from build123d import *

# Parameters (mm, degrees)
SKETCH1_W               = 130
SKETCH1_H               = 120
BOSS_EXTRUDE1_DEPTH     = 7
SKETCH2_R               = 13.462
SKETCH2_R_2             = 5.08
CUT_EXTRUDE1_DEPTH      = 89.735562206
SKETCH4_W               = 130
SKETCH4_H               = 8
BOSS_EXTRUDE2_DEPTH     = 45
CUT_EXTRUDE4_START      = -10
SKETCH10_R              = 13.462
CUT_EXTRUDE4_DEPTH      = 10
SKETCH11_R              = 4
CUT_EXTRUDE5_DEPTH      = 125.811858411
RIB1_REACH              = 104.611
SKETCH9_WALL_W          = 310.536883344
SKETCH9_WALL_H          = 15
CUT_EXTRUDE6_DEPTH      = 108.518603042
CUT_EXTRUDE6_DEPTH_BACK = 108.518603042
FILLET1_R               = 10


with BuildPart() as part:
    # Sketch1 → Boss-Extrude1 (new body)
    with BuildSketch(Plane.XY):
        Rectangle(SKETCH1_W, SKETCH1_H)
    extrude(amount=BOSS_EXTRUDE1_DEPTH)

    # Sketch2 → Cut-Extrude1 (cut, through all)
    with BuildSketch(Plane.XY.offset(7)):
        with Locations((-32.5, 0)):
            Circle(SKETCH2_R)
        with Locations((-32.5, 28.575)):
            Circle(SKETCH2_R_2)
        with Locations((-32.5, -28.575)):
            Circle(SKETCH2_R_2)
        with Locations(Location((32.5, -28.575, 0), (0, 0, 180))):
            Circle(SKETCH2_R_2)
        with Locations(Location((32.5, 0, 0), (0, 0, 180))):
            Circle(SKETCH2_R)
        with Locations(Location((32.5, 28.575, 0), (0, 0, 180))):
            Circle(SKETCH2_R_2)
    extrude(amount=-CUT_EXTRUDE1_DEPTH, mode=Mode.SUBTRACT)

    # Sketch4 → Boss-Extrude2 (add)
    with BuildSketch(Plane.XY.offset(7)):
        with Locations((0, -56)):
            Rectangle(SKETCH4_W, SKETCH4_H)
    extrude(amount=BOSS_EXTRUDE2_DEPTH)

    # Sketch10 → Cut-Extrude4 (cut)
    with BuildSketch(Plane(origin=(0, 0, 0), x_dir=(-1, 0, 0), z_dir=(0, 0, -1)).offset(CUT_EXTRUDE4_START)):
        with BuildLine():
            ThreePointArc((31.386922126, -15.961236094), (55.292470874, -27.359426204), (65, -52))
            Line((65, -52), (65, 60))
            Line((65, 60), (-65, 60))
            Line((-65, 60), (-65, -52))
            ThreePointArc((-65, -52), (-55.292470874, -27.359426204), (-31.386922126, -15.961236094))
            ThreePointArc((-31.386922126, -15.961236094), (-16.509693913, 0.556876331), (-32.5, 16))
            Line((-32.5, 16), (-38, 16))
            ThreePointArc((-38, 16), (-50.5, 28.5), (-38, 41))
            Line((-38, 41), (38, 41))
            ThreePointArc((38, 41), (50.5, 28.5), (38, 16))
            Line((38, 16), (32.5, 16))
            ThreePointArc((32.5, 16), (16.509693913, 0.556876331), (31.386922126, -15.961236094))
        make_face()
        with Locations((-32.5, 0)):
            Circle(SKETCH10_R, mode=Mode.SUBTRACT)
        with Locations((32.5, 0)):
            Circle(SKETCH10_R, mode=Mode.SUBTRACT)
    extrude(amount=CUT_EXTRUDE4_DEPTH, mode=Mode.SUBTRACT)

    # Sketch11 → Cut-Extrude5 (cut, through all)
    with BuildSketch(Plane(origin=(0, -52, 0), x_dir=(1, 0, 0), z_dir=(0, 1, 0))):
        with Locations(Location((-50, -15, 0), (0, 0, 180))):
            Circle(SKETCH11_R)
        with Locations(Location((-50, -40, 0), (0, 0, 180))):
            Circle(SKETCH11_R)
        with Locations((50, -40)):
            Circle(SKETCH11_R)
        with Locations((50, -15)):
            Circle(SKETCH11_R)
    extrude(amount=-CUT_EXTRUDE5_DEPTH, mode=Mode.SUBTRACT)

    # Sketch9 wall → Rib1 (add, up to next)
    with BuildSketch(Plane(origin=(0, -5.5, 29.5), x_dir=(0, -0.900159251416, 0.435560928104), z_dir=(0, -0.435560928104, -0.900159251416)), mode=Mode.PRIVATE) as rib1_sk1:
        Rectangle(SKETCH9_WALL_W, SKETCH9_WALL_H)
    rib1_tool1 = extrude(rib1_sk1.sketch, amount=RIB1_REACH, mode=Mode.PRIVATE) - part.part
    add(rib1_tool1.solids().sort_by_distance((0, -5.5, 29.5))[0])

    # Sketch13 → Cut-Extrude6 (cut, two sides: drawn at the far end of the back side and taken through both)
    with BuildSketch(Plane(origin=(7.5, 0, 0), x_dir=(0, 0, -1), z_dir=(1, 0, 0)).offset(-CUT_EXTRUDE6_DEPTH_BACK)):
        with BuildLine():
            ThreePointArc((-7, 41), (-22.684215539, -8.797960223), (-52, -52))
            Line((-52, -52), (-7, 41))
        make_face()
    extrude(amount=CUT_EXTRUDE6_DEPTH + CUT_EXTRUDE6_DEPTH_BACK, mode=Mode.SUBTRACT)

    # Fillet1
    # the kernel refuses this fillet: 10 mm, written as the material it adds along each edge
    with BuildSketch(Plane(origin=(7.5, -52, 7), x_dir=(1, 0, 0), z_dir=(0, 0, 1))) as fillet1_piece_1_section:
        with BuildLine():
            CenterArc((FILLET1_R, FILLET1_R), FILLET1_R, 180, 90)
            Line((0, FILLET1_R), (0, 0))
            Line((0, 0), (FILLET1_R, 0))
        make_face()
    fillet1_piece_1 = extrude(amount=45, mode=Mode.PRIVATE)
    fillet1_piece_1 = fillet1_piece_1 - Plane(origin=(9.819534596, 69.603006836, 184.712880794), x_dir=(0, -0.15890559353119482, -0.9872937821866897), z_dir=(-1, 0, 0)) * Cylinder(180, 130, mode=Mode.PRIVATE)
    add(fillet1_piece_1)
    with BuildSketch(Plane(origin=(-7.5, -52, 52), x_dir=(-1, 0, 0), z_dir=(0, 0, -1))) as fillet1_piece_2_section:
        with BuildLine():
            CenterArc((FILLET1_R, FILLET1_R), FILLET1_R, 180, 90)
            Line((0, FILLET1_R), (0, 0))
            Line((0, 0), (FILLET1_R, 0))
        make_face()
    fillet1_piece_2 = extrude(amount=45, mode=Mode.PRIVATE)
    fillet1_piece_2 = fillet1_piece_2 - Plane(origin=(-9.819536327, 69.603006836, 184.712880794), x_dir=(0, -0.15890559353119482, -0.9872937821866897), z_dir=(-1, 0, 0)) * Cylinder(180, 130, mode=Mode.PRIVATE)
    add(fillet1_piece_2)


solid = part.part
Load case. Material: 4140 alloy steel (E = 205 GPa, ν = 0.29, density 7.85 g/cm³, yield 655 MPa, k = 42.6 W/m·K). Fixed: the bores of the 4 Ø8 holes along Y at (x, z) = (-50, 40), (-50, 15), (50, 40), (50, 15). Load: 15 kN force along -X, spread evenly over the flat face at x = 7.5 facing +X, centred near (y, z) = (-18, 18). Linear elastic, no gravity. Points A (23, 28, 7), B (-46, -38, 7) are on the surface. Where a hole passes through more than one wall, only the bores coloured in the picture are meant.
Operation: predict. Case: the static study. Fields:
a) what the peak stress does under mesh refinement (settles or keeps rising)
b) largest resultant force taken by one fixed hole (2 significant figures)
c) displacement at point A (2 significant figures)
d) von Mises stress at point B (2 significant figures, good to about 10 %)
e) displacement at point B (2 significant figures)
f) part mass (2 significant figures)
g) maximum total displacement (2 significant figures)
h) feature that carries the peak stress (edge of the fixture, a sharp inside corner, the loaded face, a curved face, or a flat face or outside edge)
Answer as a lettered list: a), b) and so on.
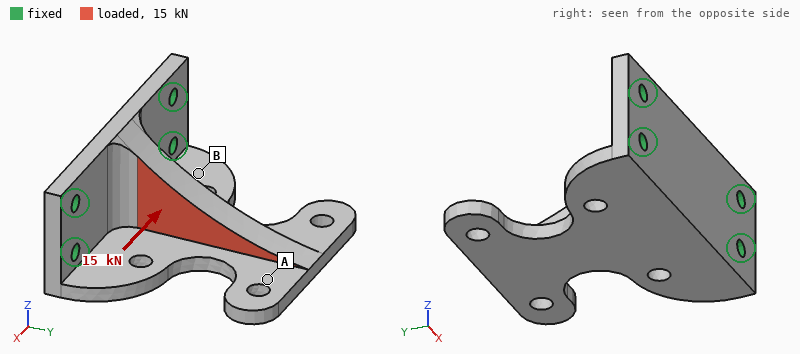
a) keeps rising
b) 7.7 kN
c) 0.066 mm
d) 28 MPa
e) 0.018 mm
f) 1.0 kg
g) 0.10 mm
h) edge of the fixture
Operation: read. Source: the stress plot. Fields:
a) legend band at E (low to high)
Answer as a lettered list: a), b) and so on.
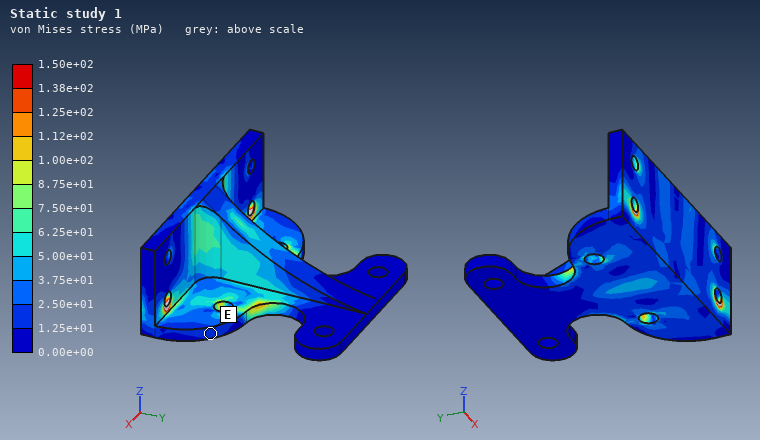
a) 1.25e+01 to 2.50e+01 MPa
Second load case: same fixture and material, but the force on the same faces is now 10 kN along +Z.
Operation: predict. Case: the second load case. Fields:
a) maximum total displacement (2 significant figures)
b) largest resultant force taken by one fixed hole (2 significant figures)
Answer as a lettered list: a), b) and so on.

a) 0.37 mm
b) 7.6 kN
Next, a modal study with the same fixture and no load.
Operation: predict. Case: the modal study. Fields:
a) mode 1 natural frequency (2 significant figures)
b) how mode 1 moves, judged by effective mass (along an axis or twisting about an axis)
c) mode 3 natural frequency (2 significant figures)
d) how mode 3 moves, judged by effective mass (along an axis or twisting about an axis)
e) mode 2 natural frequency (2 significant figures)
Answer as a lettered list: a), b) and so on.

a) 1300 Hz
b) along Z
c) 3000 Hz
d) along X
e) 2000 Hz
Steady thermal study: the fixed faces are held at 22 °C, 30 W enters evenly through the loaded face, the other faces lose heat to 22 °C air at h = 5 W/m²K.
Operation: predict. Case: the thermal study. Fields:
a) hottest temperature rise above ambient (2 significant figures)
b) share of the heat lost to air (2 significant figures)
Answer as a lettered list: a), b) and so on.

a) 47 K
b) 13 %
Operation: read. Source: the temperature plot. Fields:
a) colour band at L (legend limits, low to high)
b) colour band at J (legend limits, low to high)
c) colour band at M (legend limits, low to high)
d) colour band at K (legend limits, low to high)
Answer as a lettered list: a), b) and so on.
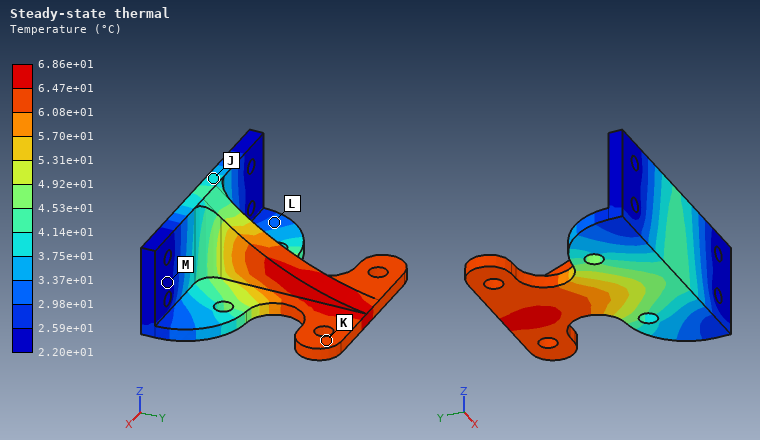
a) 2.98e+01 to 3.37e+01 °C
b) 3.75e+01 to 4.14e+01 °C
c) 2.20e+01 to 2.59e+01 °C
d) 6.08e+01 to 6.47e+01 °C
